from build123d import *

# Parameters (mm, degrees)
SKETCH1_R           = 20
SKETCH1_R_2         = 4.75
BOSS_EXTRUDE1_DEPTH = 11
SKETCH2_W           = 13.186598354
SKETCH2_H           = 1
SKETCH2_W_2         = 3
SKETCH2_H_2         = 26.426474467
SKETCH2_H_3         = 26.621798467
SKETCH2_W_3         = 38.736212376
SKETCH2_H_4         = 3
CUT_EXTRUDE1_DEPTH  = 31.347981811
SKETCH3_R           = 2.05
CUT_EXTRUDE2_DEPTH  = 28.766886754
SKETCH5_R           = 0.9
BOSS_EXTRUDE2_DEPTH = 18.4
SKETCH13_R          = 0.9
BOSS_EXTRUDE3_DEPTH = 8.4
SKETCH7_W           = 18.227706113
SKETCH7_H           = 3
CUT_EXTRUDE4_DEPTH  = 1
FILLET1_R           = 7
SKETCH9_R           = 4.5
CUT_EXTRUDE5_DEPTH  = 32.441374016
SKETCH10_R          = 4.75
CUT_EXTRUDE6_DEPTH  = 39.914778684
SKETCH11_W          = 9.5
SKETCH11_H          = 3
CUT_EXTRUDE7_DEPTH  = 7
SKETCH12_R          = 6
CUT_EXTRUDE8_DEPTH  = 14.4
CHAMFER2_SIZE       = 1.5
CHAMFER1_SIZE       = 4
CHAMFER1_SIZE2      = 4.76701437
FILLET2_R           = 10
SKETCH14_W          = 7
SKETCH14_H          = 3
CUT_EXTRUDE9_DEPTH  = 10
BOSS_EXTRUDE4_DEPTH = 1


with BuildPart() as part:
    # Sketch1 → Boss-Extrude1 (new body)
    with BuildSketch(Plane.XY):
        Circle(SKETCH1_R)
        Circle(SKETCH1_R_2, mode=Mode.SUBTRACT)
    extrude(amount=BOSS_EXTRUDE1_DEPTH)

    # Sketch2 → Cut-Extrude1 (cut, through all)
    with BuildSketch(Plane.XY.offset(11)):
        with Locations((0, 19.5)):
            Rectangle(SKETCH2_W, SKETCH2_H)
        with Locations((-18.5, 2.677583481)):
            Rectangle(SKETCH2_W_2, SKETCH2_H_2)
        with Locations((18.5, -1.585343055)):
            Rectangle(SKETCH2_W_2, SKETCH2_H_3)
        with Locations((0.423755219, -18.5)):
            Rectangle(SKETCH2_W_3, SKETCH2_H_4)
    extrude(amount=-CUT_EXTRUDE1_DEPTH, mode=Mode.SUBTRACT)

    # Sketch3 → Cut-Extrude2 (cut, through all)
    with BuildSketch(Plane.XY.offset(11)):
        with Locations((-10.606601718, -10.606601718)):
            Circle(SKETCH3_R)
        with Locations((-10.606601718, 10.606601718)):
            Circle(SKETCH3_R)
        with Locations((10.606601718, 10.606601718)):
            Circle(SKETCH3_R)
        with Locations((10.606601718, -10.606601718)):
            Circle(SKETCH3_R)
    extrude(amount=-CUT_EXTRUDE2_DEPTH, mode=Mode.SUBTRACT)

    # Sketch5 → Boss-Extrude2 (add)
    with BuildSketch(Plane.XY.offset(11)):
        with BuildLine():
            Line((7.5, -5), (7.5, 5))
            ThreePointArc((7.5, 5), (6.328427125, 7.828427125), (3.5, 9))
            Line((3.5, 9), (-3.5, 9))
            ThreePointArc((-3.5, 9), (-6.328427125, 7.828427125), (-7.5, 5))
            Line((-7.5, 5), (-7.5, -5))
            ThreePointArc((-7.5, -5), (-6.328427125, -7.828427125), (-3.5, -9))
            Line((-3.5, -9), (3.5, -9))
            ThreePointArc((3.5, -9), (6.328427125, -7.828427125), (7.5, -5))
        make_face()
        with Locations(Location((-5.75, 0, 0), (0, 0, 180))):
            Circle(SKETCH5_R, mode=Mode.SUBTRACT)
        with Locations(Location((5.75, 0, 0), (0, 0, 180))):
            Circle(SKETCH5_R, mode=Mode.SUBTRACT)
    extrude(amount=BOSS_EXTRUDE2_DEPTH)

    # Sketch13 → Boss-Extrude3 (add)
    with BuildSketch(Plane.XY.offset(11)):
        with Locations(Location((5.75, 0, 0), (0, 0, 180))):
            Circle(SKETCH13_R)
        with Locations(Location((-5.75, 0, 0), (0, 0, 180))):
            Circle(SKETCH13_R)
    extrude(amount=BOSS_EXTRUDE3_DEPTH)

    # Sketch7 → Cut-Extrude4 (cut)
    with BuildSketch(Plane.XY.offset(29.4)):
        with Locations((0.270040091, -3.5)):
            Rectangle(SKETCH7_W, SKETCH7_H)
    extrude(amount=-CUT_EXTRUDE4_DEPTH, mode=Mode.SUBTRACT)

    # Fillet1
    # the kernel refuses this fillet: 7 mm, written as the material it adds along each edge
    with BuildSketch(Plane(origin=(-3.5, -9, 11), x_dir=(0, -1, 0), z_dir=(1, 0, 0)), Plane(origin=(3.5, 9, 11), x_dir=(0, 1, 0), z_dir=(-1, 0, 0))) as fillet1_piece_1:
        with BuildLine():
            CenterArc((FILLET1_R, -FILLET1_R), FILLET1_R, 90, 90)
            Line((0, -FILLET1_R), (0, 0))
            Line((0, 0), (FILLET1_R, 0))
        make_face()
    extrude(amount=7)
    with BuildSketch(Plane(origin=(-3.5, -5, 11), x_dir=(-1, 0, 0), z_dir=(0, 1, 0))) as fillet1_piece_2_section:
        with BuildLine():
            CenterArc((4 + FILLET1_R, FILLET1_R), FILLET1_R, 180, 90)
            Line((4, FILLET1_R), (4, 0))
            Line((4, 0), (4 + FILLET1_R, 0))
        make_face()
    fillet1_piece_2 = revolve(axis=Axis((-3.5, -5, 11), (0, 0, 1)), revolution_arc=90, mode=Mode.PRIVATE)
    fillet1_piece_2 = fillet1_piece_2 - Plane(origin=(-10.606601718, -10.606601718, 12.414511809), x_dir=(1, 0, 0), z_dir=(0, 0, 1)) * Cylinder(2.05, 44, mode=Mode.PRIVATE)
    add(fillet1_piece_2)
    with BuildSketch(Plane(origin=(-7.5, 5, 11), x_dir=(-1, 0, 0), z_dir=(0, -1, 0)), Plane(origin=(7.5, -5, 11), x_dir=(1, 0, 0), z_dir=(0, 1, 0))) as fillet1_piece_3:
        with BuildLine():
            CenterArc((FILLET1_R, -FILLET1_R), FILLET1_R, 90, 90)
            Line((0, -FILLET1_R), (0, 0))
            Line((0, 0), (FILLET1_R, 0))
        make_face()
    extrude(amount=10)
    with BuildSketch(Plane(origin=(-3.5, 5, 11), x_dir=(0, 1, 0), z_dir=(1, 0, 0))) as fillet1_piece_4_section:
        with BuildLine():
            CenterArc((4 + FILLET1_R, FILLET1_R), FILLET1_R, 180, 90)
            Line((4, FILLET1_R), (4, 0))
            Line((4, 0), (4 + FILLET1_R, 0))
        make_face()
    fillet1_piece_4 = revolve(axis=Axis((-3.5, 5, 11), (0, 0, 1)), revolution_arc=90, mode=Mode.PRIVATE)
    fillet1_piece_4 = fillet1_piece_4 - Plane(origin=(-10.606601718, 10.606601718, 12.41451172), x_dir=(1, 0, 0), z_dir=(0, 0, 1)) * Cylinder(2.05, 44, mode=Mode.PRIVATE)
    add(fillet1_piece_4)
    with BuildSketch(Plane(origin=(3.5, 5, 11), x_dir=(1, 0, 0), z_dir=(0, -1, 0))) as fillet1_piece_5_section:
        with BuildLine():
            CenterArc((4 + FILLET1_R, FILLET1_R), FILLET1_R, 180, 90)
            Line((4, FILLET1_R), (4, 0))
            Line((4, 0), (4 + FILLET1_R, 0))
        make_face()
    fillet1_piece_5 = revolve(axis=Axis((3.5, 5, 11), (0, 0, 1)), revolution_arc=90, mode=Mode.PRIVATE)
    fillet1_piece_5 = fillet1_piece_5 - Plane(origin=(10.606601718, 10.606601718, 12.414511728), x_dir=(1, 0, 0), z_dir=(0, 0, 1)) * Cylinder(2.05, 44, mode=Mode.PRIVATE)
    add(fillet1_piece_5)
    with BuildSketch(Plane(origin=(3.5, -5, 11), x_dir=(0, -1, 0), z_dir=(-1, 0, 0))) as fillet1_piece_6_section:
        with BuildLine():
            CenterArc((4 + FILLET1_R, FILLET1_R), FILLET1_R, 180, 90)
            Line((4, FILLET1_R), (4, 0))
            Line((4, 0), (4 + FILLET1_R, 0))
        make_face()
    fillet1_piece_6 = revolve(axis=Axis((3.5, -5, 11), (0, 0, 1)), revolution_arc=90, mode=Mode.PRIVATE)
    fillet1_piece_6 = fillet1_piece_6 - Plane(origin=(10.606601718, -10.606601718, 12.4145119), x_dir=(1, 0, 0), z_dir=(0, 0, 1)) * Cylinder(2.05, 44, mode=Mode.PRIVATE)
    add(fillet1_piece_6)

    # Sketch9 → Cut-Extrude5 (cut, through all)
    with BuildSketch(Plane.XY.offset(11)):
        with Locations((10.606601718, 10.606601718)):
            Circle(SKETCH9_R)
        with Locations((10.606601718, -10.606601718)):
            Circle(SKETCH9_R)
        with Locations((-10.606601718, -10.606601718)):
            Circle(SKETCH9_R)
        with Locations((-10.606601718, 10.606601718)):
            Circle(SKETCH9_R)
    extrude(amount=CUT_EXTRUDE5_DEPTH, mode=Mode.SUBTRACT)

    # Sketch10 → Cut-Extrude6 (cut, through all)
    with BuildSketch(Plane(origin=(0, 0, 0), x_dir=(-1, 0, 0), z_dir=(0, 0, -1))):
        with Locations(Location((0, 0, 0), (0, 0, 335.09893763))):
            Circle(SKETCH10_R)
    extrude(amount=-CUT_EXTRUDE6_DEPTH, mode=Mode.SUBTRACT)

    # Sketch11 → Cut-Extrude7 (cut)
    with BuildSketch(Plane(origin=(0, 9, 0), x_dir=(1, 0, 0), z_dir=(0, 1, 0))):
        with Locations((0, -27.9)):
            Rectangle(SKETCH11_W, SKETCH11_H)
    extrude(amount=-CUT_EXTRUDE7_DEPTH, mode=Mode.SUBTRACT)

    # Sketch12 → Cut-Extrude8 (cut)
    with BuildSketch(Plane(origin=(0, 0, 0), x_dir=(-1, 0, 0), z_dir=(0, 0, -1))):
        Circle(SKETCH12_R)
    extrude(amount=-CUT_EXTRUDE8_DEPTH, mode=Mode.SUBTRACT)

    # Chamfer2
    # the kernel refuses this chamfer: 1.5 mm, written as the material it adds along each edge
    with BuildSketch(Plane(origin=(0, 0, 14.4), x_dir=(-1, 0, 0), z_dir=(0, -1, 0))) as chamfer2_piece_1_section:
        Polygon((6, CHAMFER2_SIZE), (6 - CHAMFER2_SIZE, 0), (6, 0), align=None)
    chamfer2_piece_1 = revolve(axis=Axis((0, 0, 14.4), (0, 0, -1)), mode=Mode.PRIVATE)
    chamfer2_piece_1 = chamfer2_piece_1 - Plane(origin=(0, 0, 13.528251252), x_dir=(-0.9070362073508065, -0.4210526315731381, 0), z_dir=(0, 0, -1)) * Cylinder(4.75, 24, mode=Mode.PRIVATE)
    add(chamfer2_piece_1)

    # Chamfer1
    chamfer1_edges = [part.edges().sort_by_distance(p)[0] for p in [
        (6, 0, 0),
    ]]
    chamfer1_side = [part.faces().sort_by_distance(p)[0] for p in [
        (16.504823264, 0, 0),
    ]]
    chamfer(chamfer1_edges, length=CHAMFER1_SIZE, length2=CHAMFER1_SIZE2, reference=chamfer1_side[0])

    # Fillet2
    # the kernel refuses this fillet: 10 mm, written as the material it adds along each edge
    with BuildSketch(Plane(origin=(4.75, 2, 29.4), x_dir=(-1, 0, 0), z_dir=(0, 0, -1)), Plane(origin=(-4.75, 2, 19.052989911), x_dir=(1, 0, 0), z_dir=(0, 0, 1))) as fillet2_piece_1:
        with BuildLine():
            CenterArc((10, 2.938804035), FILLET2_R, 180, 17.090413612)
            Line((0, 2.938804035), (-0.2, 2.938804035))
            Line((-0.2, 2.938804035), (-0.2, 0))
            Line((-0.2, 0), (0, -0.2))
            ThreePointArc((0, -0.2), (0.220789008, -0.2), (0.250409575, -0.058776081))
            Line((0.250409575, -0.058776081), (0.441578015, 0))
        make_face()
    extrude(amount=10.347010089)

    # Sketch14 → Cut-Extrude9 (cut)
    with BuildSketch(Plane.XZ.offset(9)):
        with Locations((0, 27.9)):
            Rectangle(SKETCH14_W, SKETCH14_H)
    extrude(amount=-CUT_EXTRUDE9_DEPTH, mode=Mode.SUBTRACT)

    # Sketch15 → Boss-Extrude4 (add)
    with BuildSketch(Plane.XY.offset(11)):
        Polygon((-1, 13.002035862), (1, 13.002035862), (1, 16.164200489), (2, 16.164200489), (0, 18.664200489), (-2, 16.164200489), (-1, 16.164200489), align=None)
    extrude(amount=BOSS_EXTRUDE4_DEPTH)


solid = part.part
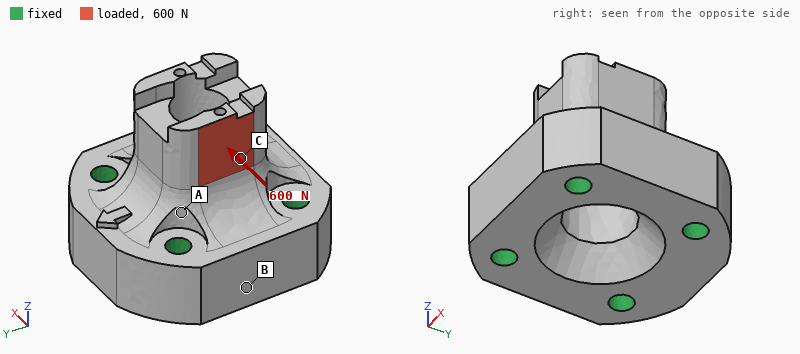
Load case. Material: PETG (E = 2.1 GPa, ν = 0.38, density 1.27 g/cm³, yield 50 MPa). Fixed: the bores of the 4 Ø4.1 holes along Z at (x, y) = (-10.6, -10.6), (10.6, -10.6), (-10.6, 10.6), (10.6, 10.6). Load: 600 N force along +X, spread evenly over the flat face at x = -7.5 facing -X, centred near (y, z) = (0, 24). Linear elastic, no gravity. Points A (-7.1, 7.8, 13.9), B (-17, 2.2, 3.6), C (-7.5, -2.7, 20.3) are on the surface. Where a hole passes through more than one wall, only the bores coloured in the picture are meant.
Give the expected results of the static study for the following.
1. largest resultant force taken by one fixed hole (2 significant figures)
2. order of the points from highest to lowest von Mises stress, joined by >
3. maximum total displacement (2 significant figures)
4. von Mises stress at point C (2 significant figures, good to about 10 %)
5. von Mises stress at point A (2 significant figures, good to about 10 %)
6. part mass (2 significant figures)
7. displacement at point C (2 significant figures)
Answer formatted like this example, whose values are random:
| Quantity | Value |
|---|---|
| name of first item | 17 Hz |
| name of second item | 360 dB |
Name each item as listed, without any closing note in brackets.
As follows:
| Quantity | Value |
|---|---|
| largest resultant force taken by one fixed hole | 290 N |
| order of the points from highest to lowest von Mises stress, joined by > | C > A > B |
| maximum total displacement | 0.39 mm |
| von Mises stress at point C | 11 MPa |
| von Mises stress at point A | 6.5 MPa |
| part mass | 17 g |
| displacement at point C | 0.15 mm |
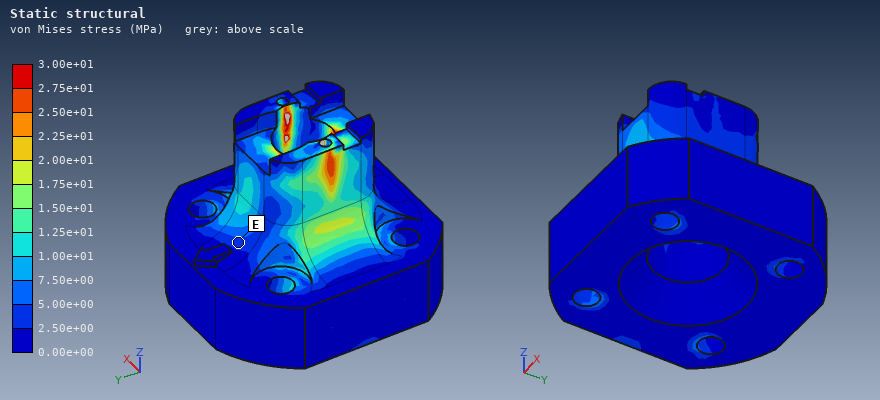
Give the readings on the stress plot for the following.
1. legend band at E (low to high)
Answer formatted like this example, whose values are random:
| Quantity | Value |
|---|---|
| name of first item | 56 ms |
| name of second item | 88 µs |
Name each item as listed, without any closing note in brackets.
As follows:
| Quantity | Value |
|---|---|
| legend band at E | 2.50e+00 to 5.00e+00 MPa |
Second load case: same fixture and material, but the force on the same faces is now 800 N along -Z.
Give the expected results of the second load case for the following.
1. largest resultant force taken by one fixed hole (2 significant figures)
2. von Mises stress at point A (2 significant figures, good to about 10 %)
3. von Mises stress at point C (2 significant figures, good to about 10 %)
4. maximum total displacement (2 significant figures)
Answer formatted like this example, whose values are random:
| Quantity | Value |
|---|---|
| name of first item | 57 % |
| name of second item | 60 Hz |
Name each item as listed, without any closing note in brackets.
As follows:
| Quantity | Value |
|---|---|
| largest resultant force taken by one fixed hole | 380 N |
| von Mises stress at point A | 9.0 MPa |
| von Mises stress at point C | 25 MPa |
| maximum total displacement | 0.36 mm |
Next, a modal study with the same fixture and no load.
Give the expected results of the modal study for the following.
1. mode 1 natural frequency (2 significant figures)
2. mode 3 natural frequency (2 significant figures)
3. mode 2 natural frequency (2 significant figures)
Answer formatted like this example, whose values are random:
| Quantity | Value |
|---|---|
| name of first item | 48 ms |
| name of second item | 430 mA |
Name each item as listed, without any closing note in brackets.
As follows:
| Quantity | Value |
|---|---|
| mode 1 natural frequency | 6900 Hz |
| mode 3 natural frequency | 11 kHz |
| mode 2 natural frequency | 7100 Hz |
